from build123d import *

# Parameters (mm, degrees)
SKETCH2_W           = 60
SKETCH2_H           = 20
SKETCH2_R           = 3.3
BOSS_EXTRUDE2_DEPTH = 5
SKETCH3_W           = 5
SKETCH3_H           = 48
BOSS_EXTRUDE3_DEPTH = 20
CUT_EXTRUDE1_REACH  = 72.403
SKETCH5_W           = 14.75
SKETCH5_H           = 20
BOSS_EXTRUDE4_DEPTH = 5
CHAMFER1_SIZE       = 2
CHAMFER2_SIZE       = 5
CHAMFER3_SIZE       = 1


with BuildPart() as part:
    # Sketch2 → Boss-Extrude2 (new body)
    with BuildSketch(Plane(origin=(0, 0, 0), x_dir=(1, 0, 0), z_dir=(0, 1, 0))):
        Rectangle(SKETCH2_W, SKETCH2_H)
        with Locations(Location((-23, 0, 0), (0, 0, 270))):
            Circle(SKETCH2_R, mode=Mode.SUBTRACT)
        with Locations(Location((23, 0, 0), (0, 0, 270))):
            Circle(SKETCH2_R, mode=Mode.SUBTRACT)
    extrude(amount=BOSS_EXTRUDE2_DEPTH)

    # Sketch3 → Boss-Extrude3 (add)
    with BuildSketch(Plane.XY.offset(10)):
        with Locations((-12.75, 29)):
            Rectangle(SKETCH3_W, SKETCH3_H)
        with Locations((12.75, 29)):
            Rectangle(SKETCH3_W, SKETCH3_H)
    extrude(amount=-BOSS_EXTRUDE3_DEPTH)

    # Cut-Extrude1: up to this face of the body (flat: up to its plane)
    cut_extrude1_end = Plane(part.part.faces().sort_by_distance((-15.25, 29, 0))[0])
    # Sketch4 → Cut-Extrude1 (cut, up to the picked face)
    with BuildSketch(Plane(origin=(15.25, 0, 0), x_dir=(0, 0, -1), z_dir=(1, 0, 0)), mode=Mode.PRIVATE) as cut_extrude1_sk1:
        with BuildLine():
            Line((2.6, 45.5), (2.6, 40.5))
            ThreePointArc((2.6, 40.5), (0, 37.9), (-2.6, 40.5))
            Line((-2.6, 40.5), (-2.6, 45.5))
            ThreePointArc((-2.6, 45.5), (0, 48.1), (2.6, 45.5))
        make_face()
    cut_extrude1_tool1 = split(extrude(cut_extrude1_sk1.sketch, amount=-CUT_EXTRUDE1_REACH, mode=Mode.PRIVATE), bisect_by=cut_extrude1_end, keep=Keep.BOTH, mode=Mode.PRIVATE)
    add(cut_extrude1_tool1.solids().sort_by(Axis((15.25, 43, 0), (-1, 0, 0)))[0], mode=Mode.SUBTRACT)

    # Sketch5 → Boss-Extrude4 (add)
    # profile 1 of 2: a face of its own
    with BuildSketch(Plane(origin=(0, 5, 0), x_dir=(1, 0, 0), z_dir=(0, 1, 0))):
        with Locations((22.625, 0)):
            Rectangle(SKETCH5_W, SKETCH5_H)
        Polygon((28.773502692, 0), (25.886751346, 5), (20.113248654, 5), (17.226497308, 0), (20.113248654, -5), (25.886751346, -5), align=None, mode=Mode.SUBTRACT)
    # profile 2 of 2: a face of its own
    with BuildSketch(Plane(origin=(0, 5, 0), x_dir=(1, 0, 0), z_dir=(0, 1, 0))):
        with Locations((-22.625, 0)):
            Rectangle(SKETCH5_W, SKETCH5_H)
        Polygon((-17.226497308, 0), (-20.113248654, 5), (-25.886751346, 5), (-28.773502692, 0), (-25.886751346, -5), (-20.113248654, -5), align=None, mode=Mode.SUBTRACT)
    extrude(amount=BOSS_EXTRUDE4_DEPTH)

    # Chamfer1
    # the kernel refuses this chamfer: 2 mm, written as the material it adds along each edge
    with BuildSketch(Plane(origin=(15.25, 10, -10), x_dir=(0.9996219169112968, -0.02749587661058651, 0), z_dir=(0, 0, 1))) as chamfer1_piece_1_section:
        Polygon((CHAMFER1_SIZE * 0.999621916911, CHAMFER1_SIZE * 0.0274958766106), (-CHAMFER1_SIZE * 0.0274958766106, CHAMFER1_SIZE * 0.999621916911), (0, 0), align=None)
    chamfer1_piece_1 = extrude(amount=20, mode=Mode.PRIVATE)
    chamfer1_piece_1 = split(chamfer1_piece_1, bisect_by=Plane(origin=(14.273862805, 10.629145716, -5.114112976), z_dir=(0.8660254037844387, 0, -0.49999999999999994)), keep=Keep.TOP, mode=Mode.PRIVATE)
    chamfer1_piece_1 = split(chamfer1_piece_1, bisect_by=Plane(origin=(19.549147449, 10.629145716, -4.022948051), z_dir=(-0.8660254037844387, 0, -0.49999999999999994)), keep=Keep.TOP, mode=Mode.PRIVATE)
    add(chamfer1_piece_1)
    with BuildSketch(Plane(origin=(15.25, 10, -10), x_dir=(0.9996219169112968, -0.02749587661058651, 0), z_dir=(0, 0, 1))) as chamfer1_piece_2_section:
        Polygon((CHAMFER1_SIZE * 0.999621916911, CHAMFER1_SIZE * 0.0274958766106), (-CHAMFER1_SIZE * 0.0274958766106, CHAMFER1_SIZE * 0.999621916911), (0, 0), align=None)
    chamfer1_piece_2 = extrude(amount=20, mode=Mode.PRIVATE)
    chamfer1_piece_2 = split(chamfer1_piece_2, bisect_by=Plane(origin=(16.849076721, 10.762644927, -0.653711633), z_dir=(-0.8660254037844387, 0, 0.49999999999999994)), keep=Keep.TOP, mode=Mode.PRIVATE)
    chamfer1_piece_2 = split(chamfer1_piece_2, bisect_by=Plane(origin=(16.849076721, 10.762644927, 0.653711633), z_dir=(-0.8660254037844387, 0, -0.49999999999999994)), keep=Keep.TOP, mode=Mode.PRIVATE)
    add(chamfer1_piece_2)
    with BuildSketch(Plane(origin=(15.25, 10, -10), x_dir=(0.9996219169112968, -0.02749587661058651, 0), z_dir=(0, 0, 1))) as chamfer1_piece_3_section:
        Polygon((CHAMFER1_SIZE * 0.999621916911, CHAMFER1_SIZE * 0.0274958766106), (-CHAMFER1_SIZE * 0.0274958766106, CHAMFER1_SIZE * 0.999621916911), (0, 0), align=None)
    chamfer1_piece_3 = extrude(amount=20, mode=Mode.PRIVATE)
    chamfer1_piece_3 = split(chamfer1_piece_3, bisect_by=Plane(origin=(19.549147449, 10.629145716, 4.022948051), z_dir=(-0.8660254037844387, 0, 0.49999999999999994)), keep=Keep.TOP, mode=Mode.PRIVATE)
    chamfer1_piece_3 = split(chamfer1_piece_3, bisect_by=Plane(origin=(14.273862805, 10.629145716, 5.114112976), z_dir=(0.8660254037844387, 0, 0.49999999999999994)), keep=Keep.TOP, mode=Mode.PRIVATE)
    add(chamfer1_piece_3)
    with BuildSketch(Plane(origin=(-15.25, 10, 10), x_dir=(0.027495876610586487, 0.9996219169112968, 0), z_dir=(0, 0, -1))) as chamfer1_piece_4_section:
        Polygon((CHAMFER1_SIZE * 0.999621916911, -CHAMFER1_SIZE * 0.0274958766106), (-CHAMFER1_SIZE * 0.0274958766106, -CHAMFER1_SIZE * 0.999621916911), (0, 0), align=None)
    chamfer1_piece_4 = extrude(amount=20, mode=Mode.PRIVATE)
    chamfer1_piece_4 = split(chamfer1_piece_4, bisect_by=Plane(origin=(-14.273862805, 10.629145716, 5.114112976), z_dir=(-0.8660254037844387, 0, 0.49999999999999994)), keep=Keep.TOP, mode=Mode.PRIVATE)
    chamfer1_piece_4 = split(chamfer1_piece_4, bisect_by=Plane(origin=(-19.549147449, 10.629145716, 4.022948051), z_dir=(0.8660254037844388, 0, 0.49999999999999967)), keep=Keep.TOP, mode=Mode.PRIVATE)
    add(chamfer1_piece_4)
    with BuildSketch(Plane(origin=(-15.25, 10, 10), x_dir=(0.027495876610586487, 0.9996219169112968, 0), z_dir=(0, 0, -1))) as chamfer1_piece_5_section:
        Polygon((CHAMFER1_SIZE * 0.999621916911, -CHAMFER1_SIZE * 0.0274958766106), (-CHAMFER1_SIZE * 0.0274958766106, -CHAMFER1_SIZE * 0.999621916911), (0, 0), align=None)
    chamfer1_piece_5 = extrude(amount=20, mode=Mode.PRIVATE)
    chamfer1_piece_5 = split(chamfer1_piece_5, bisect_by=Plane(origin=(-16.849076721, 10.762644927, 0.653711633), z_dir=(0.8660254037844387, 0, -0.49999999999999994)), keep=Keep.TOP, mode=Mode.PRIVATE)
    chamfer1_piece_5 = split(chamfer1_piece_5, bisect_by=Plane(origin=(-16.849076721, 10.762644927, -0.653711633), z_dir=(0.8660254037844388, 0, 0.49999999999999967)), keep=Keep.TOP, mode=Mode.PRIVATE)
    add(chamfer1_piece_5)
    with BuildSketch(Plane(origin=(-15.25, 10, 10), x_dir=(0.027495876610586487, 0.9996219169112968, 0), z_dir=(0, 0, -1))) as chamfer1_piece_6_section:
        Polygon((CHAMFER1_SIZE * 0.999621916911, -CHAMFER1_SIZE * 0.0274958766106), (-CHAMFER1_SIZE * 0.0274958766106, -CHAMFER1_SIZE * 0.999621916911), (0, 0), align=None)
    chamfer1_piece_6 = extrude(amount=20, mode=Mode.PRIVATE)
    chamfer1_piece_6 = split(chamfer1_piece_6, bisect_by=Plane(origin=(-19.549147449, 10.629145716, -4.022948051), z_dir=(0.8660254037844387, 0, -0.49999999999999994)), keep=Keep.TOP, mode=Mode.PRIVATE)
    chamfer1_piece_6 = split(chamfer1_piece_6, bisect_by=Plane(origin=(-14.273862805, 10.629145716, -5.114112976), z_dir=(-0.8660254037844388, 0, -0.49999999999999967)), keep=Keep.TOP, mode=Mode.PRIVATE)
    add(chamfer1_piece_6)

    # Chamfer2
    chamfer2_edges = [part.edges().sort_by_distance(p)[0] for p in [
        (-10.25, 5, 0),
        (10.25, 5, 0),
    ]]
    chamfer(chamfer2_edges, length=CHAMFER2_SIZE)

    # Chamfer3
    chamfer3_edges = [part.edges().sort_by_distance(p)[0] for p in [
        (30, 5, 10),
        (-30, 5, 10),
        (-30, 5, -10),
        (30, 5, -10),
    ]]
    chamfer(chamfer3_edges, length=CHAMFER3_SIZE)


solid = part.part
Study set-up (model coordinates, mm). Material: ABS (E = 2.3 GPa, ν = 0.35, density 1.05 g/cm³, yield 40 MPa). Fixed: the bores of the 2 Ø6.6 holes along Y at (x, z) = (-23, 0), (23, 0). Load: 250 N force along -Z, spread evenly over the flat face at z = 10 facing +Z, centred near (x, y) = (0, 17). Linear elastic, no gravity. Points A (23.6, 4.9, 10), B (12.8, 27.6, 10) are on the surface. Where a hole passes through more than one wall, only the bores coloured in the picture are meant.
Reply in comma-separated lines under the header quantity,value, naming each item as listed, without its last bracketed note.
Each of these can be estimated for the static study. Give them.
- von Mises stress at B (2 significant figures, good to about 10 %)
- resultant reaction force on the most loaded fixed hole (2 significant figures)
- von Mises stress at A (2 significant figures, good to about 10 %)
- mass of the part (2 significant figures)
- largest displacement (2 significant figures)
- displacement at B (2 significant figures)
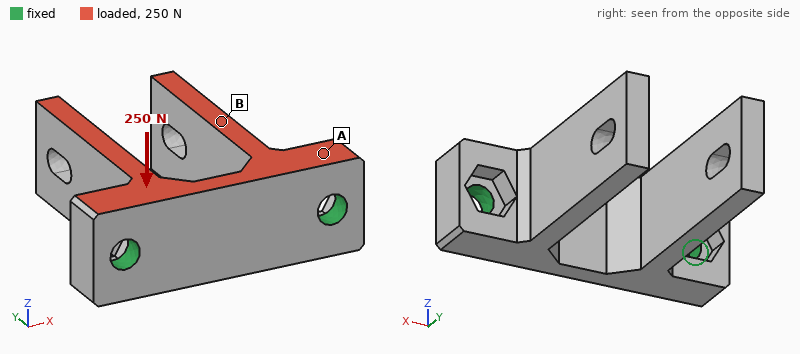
quantity,value
von Mises stress at B,1.5 MPa
resultant reaction force on the most loaded fixed hole,130 N
von Mises stress at A,3.4 MPa
mass of the part,18 g
largest displacement,0.49 mm
displacement at B,0.24 mm
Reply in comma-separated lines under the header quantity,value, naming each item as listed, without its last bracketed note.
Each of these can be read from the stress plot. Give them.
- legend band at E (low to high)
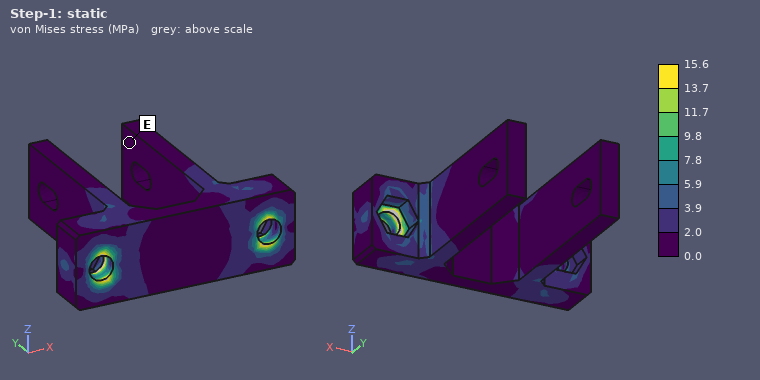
quantity,value
legend band at E,0.0 to 2.0 MPa
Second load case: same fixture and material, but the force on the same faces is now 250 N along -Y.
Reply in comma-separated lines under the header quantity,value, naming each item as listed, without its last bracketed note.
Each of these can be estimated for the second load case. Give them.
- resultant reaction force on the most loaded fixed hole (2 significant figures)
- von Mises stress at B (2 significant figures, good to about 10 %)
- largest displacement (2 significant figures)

quantity,value
resultant reaction force on the most loaded fixed hole,130 N
von Mises stress at B,1.5 MPa
largest displacement,0.35 mm
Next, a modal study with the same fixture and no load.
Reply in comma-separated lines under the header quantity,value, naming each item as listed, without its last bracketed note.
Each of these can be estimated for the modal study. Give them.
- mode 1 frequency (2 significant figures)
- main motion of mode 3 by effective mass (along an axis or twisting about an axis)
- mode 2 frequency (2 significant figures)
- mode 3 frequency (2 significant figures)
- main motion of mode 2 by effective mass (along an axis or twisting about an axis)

quantity,value
mode 1 frequency,590 Hz
main motion of mode 3 by effective mass,along Z
mode 2 frequency,640 Hz
mode 3 frequency,1100 Hz
main motion of mode 2 by effective mass,along X
